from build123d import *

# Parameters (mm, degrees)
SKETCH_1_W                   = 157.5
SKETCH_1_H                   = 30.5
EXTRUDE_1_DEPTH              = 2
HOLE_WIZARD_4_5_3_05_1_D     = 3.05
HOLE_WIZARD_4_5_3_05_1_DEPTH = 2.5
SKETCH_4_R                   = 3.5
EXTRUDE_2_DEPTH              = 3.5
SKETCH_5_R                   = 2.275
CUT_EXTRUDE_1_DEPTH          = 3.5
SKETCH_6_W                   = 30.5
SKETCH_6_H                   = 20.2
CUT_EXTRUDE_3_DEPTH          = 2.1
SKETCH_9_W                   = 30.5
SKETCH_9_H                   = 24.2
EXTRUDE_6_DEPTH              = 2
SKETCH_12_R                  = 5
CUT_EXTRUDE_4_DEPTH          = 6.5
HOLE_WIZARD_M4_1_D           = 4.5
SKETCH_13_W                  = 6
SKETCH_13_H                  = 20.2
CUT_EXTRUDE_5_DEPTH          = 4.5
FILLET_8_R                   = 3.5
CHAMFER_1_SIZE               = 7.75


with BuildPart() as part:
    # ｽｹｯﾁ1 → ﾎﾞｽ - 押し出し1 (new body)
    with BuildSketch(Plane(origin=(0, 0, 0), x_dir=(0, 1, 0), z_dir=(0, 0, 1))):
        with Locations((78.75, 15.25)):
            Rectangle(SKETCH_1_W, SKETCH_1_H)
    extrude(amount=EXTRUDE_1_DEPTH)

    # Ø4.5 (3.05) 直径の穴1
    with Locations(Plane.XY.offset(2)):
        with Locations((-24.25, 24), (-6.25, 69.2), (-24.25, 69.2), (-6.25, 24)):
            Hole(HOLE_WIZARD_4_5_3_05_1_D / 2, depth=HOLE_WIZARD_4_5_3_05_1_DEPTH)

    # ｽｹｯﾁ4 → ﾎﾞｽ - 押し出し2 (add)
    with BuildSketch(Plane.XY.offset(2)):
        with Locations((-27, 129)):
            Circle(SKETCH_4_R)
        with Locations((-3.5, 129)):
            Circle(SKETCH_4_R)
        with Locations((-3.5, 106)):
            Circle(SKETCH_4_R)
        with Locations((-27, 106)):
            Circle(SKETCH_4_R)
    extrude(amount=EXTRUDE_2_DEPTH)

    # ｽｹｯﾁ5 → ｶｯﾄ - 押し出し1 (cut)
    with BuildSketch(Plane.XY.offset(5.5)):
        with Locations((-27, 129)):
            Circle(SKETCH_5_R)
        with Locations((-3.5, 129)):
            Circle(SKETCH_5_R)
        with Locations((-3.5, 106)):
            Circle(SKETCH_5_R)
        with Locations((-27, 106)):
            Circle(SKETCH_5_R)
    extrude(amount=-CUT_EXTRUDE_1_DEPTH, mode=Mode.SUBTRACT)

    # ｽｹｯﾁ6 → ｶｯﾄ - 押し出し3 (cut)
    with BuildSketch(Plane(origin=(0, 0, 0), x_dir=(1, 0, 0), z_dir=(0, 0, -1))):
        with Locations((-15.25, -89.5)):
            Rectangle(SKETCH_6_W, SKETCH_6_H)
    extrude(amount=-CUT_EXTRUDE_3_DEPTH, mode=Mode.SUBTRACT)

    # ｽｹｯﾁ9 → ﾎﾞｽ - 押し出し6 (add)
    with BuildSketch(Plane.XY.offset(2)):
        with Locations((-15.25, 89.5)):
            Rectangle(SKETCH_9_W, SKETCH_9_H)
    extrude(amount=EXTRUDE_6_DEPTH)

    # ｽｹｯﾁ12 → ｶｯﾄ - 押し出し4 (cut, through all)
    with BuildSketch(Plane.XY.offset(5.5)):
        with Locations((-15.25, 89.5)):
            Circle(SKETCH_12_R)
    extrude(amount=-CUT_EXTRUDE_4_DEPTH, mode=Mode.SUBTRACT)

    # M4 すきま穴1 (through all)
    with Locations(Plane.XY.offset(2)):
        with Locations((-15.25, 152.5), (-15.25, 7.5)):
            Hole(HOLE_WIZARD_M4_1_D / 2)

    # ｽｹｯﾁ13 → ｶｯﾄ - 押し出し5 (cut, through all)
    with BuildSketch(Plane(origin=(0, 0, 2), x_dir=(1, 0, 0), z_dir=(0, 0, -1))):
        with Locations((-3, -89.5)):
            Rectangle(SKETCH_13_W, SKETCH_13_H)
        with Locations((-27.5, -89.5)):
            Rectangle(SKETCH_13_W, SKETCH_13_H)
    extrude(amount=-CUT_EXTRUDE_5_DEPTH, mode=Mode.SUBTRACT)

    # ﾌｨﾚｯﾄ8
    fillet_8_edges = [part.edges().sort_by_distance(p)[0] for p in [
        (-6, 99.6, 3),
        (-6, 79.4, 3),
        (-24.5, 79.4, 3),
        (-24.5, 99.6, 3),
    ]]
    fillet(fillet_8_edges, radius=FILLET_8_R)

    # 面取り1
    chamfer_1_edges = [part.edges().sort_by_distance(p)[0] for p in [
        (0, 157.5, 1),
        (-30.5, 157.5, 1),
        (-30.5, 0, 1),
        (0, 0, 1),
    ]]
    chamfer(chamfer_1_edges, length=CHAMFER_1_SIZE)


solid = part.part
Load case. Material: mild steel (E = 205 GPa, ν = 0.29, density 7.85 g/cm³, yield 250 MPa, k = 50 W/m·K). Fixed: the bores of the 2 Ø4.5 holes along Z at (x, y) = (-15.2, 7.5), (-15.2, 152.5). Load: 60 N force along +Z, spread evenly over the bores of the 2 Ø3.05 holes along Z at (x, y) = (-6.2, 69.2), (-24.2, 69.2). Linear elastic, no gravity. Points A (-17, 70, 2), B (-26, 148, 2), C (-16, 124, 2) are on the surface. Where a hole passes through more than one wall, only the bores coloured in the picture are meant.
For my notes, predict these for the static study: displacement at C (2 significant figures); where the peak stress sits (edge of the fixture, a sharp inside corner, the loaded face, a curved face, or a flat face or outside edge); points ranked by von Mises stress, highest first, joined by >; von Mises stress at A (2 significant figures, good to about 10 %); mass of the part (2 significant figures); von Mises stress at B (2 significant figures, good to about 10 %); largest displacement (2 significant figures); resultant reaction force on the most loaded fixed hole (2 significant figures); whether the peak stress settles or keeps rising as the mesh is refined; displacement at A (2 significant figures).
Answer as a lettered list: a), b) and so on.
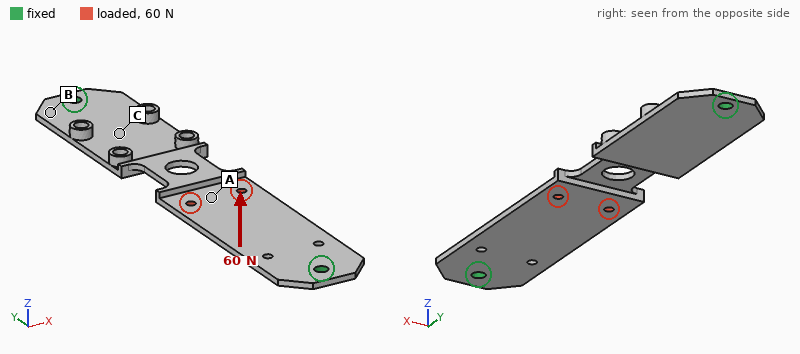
a) 0.063 mm
b) edge of the fixture
c) A > B > C
d) 58 MPa
e) 72 g
f) 25 MPa
g) 0.21 mm
h) 230 N
i) keeps rising
j) 0.21 mm
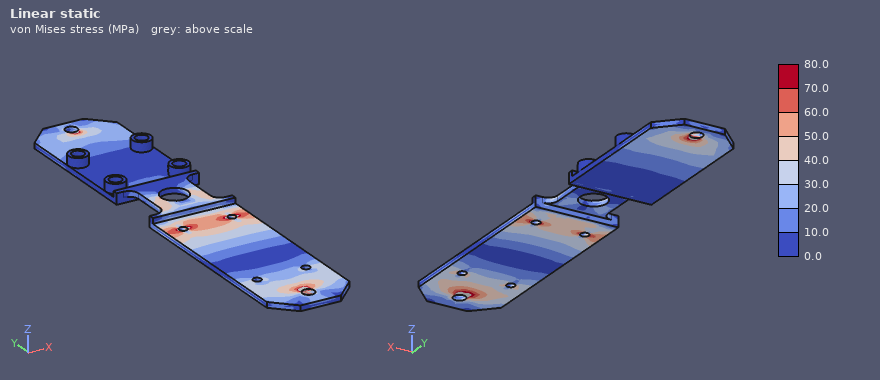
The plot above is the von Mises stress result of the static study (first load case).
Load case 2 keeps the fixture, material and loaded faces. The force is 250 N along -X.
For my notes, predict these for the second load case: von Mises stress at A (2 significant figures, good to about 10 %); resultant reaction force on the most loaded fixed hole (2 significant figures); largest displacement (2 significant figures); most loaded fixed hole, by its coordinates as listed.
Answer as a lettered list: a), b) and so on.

a) 9.6 MPa
b) 150 N
c) 32 µm
d) (-15.2, 7.5)
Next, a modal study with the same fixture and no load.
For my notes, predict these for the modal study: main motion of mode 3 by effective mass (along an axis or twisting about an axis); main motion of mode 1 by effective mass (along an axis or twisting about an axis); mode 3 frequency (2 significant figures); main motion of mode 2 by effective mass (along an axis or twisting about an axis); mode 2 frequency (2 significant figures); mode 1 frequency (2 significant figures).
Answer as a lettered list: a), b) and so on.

a) twisting about Y
b) along Z
c) 1500 Hz
d) twisting about X
e) 1300 Hz
f) 530 Hz
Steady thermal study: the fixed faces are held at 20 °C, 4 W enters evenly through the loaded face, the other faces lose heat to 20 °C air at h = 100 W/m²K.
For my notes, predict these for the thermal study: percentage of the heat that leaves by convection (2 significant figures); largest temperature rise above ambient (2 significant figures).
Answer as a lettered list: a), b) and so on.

a) 94 %
b) 18 K
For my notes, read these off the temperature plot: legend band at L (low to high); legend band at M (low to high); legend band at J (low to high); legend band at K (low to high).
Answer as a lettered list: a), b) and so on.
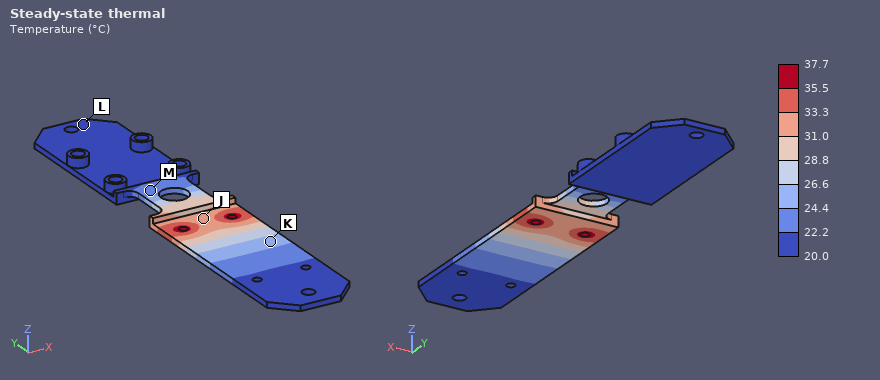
a) 20.0 to 22.2 °C
b) 22.2 to 24.4 °C
c) 31.0 to 33.3 °C
d) 24.4 to 26.6 °C
